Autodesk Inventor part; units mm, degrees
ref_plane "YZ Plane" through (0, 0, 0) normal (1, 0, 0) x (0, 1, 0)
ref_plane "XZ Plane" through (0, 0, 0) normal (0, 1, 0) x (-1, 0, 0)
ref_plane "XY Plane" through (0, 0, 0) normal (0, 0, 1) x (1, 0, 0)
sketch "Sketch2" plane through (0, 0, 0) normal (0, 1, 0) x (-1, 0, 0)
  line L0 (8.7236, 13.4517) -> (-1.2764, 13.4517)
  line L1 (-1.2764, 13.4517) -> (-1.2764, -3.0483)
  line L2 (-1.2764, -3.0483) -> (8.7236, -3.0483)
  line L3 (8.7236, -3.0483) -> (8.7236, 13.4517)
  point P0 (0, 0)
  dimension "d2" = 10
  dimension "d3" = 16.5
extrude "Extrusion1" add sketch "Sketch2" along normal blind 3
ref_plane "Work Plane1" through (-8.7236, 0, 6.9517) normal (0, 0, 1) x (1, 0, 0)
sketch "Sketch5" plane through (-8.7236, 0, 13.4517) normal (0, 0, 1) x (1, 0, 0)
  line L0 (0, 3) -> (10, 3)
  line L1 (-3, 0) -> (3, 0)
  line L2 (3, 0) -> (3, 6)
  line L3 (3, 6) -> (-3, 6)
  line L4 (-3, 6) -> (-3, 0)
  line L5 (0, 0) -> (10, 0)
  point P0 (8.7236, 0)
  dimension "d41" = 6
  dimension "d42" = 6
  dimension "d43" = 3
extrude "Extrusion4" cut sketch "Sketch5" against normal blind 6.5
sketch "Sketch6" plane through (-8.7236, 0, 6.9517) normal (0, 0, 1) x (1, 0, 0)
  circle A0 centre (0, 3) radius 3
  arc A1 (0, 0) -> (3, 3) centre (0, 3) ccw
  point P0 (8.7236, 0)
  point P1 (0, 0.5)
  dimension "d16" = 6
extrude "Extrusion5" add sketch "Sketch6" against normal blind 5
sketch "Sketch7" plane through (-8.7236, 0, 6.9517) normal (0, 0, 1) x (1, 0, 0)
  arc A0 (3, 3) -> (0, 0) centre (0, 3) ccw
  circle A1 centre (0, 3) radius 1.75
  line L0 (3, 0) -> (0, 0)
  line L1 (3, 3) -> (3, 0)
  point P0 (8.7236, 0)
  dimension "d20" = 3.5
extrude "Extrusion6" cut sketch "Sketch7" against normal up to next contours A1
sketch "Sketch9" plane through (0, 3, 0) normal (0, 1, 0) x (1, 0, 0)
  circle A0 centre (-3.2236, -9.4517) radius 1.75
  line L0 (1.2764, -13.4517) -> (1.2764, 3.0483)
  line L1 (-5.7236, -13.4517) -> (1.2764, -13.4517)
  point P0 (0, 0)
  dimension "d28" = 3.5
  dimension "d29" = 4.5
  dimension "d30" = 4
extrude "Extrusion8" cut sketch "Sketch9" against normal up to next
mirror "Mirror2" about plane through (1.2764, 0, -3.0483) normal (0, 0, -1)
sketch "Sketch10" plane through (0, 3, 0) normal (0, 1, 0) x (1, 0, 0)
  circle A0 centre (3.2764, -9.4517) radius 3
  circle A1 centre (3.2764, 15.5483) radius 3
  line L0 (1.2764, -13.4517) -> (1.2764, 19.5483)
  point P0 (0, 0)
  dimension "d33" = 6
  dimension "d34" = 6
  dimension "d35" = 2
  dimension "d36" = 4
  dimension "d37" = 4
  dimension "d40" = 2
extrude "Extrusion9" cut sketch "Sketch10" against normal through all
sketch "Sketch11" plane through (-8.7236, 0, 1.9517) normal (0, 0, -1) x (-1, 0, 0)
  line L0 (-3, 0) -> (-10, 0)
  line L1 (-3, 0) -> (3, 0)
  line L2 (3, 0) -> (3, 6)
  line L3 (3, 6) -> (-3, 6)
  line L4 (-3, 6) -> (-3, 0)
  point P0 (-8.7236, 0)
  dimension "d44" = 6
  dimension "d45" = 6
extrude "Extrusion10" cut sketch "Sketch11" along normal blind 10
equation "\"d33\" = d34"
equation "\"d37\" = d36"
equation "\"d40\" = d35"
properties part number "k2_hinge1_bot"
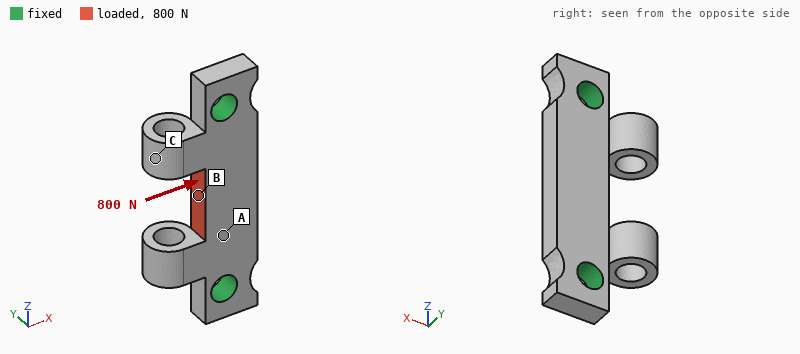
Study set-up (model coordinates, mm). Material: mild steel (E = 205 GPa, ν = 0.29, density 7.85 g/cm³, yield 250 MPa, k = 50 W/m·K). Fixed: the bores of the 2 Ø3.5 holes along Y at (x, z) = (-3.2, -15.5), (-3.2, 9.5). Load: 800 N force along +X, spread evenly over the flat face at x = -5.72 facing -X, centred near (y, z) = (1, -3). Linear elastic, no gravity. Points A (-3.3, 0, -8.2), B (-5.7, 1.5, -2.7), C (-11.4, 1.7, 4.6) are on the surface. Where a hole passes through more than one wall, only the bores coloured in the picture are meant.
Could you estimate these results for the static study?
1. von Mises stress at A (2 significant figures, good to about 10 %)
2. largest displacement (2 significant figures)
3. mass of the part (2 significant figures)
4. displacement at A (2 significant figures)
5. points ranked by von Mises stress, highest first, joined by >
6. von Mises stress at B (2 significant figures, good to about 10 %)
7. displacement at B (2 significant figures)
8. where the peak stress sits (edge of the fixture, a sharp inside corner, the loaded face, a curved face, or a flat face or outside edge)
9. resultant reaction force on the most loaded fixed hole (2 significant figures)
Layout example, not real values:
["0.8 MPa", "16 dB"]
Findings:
["45 MPa", "6.9 µm", "6.5 g", "4.2 µm", "B > A > C", "66 MPa", "6.2 µm", "edge of the fixture", "410 N"]
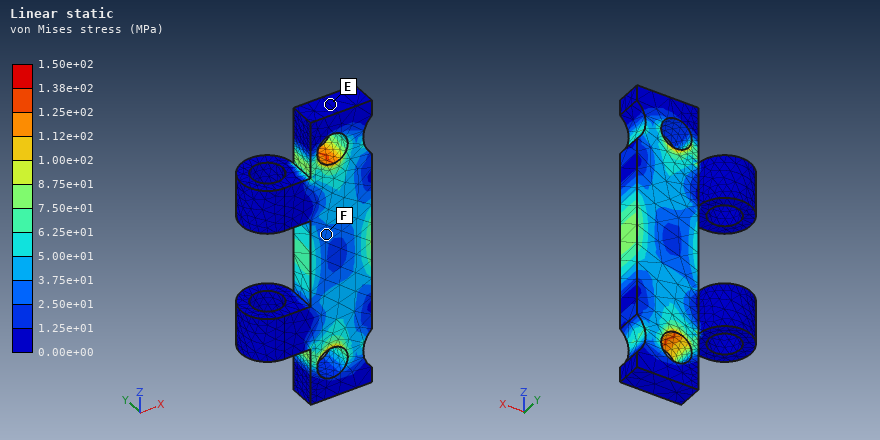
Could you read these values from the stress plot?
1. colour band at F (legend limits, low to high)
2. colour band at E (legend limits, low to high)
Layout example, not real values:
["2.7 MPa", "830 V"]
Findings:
["2.50e+01 to 3.75e+01 MPa", "0.00e+00 to 1.25e+01 MPa"]
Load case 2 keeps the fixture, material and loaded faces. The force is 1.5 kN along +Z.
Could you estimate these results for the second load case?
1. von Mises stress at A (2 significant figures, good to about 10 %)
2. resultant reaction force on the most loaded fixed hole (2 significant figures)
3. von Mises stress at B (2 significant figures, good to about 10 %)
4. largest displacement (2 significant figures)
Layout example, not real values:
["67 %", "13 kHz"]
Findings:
["44 MPa", "780 N", "88 MPa", "3.3 µm"]
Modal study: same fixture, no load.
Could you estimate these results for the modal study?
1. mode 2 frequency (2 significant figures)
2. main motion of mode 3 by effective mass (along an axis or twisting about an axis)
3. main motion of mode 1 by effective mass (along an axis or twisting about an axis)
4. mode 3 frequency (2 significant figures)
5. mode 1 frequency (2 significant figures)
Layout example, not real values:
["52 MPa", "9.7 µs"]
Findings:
["23 kHz", "along Y", "along Y", "26 kHz", "21 kHz"]
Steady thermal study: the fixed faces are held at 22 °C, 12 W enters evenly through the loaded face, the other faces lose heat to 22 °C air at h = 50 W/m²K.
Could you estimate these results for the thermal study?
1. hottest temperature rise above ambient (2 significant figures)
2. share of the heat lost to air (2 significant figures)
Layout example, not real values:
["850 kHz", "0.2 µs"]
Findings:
["62 K", "7.4 %"]
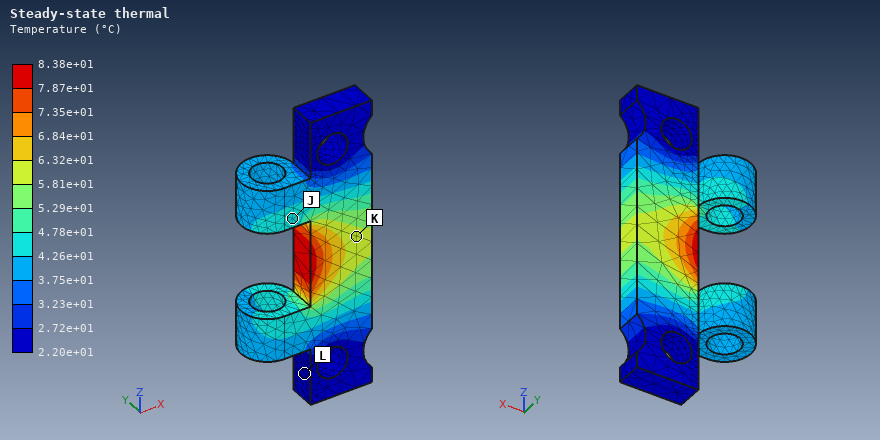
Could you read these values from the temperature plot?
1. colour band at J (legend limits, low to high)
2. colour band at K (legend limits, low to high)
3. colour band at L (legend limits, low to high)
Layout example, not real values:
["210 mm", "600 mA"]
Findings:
["4.26e+01 to 4.78e+01 °C", "5.81e+01 to 6.32e+01 °C", "2.20e+01 to 2.72e+01 °C"]
